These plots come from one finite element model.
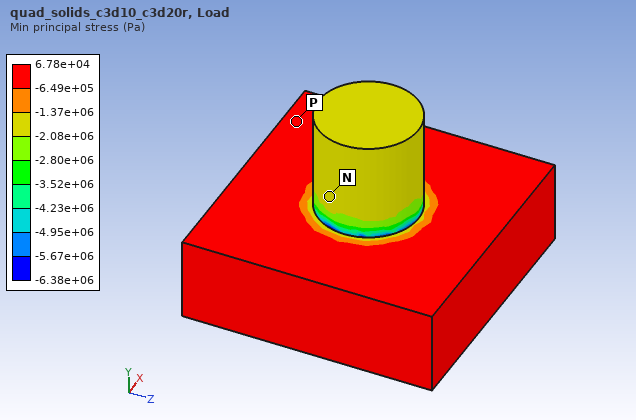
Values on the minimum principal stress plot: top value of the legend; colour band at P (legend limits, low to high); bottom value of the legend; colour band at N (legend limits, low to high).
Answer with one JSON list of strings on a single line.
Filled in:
["6.78e+04 Pa", "-6.49e+05 to 6.78e+04 Pa", "-6.38e+06 Pa", "-2.08e+06 to -1.37e+06 Pa"]
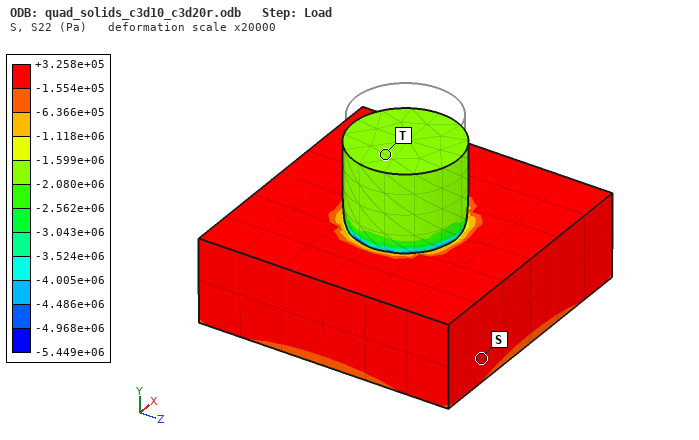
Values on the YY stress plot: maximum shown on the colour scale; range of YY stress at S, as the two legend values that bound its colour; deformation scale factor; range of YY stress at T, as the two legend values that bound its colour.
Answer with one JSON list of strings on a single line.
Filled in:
["+3.258e+05 Pa", "-1.554e+05 to +3.258e+05 Pa", "20000", "-2.080e+06 to -1.599e+06 Pa"]
